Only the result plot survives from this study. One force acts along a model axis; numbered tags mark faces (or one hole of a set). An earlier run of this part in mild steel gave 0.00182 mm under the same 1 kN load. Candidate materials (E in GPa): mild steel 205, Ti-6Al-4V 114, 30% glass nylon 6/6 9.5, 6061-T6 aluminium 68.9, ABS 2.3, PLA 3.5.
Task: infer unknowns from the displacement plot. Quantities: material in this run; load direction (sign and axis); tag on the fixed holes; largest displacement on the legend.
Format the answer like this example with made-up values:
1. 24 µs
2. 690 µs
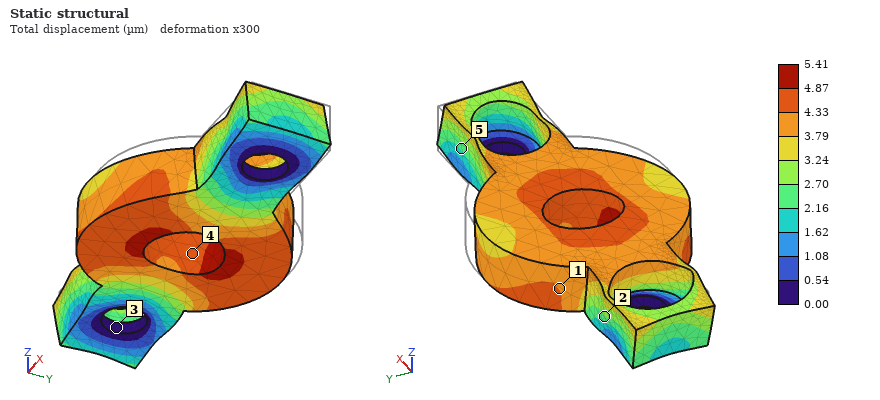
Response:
1. 6061-T6 aluminium
2. -X
3. 3
4. 5.41 µm
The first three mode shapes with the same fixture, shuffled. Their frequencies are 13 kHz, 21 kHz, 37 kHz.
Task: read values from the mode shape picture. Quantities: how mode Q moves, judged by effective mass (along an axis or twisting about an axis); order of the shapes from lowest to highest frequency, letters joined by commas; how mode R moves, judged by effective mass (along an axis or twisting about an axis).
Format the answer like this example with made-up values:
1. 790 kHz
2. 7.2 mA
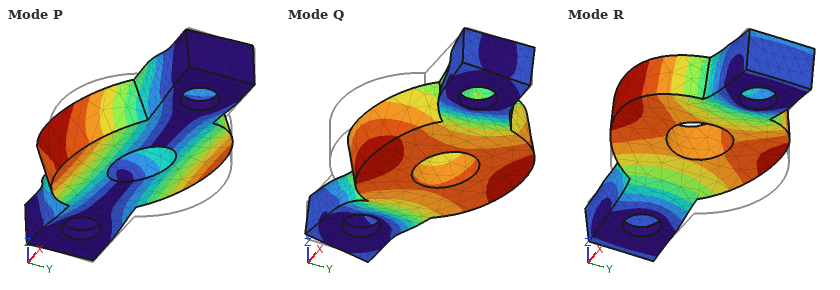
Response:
1. along Y
2. P, R, Q
3. along Z
